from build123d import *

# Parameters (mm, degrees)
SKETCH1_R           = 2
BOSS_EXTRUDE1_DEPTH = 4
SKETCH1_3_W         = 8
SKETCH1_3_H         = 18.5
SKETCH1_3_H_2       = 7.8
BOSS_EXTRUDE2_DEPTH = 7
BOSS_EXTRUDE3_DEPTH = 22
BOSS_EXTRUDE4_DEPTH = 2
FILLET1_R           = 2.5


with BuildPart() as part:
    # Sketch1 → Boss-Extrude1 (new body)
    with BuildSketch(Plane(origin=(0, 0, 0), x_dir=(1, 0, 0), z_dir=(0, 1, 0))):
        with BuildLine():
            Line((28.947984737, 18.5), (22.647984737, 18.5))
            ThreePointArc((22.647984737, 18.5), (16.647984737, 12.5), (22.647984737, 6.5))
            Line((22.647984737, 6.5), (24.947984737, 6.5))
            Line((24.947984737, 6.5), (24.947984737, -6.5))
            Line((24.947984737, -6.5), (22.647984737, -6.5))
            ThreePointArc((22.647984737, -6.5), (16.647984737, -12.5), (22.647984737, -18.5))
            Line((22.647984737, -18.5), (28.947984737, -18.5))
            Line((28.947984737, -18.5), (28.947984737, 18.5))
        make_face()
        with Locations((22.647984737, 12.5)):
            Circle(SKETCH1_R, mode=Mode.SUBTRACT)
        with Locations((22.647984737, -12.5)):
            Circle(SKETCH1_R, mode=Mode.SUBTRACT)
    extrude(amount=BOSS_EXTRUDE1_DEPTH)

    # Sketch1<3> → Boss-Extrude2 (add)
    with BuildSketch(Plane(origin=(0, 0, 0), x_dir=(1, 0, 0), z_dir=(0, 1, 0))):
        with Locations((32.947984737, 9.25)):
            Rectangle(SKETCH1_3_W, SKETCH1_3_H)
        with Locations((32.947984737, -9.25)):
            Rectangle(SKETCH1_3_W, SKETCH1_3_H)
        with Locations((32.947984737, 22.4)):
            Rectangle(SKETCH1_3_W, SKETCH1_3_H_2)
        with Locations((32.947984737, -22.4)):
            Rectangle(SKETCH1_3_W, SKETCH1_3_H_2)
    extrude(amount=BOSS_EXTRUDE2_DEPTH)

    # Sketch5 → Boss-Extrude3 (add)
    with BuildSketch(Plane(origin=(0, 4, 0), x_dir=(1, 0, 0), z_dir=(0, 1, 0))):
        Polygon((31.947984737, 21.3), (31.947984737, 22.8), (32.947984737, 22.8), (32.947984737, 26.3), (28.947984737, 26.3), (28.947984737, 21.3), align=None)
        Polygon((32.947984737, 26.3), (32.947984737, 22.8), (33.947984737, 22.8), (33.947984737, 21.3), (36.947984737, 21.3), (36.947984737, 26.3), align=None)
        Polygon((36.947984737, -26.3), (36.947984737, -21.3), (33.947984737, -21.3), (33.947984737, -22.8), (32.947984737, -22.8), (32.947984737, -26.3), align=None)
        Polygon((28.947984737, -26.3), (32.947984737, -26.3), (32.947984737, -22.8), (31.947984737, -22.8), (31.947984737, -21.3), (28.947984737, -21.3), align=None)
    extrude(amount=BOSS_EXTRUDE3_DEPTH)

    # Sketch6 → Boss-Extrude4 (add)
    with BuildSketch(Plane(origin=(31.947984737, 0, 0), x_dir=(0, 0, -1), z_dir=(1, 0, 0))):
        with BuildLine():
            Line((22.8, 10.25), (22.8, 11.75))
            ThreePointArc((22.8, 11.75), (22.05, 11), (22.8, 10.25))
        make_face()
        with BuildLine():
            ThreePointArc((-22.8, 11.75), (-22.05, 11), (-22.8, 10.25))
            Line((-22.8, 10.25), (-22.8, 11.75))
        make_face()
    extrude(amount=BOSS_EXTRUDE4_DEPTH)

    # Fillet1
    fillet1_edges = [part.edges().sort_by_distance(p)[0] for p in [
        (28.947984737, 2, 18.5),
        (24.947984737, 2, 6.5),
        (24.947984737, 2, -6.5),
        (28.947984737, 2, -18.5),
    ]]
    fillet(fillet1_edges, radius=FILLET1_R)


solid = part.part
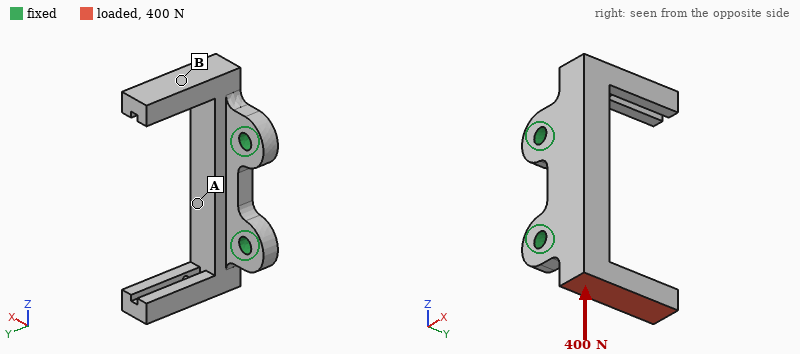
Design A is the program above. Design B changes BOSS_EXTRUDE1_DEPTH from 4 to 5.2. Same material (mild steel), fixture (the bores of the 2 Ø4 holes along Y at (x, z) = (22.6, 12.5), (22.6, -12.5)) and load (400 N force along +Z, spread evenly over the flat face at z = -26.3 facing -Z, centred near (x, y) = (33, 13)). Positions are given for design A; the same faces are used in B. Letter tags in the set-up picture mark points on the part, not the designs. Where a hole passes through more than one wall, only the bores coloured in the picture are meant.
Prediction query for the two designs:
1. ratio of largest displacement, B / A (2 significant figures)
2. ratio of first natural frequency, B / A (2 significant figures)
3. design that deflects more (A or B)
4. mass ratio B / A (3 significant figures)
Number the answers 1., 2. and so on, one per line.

1. 0.92
2. 1.3
3. A
4. 1.06
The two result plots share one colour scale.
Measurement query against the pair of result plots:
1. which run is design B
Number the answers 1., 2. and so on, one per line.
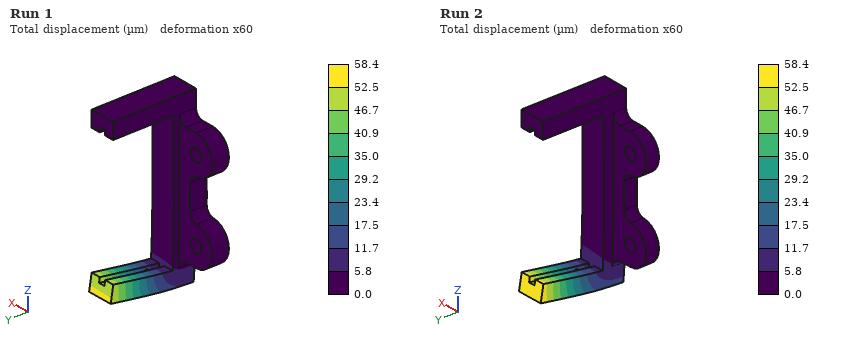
1. Run 1
